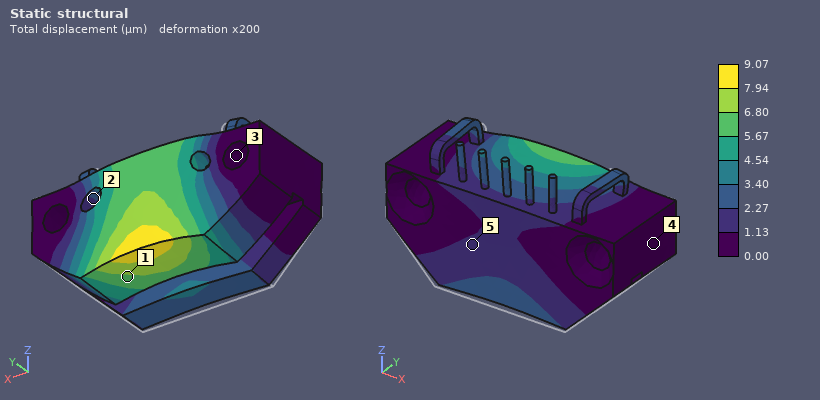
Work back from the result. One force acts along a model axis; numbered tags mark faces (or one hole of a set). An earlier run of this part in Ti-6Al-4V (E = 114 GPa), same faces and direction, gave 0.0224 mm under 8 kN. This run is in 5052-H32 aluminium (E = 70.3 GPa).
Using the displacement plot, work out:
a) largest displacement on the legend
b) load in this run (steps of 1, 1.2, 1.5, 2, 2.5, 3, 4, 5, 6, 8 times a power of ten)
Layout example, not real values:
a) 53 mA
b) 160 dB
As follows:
a) 9.07 µm
b) 2 kN
